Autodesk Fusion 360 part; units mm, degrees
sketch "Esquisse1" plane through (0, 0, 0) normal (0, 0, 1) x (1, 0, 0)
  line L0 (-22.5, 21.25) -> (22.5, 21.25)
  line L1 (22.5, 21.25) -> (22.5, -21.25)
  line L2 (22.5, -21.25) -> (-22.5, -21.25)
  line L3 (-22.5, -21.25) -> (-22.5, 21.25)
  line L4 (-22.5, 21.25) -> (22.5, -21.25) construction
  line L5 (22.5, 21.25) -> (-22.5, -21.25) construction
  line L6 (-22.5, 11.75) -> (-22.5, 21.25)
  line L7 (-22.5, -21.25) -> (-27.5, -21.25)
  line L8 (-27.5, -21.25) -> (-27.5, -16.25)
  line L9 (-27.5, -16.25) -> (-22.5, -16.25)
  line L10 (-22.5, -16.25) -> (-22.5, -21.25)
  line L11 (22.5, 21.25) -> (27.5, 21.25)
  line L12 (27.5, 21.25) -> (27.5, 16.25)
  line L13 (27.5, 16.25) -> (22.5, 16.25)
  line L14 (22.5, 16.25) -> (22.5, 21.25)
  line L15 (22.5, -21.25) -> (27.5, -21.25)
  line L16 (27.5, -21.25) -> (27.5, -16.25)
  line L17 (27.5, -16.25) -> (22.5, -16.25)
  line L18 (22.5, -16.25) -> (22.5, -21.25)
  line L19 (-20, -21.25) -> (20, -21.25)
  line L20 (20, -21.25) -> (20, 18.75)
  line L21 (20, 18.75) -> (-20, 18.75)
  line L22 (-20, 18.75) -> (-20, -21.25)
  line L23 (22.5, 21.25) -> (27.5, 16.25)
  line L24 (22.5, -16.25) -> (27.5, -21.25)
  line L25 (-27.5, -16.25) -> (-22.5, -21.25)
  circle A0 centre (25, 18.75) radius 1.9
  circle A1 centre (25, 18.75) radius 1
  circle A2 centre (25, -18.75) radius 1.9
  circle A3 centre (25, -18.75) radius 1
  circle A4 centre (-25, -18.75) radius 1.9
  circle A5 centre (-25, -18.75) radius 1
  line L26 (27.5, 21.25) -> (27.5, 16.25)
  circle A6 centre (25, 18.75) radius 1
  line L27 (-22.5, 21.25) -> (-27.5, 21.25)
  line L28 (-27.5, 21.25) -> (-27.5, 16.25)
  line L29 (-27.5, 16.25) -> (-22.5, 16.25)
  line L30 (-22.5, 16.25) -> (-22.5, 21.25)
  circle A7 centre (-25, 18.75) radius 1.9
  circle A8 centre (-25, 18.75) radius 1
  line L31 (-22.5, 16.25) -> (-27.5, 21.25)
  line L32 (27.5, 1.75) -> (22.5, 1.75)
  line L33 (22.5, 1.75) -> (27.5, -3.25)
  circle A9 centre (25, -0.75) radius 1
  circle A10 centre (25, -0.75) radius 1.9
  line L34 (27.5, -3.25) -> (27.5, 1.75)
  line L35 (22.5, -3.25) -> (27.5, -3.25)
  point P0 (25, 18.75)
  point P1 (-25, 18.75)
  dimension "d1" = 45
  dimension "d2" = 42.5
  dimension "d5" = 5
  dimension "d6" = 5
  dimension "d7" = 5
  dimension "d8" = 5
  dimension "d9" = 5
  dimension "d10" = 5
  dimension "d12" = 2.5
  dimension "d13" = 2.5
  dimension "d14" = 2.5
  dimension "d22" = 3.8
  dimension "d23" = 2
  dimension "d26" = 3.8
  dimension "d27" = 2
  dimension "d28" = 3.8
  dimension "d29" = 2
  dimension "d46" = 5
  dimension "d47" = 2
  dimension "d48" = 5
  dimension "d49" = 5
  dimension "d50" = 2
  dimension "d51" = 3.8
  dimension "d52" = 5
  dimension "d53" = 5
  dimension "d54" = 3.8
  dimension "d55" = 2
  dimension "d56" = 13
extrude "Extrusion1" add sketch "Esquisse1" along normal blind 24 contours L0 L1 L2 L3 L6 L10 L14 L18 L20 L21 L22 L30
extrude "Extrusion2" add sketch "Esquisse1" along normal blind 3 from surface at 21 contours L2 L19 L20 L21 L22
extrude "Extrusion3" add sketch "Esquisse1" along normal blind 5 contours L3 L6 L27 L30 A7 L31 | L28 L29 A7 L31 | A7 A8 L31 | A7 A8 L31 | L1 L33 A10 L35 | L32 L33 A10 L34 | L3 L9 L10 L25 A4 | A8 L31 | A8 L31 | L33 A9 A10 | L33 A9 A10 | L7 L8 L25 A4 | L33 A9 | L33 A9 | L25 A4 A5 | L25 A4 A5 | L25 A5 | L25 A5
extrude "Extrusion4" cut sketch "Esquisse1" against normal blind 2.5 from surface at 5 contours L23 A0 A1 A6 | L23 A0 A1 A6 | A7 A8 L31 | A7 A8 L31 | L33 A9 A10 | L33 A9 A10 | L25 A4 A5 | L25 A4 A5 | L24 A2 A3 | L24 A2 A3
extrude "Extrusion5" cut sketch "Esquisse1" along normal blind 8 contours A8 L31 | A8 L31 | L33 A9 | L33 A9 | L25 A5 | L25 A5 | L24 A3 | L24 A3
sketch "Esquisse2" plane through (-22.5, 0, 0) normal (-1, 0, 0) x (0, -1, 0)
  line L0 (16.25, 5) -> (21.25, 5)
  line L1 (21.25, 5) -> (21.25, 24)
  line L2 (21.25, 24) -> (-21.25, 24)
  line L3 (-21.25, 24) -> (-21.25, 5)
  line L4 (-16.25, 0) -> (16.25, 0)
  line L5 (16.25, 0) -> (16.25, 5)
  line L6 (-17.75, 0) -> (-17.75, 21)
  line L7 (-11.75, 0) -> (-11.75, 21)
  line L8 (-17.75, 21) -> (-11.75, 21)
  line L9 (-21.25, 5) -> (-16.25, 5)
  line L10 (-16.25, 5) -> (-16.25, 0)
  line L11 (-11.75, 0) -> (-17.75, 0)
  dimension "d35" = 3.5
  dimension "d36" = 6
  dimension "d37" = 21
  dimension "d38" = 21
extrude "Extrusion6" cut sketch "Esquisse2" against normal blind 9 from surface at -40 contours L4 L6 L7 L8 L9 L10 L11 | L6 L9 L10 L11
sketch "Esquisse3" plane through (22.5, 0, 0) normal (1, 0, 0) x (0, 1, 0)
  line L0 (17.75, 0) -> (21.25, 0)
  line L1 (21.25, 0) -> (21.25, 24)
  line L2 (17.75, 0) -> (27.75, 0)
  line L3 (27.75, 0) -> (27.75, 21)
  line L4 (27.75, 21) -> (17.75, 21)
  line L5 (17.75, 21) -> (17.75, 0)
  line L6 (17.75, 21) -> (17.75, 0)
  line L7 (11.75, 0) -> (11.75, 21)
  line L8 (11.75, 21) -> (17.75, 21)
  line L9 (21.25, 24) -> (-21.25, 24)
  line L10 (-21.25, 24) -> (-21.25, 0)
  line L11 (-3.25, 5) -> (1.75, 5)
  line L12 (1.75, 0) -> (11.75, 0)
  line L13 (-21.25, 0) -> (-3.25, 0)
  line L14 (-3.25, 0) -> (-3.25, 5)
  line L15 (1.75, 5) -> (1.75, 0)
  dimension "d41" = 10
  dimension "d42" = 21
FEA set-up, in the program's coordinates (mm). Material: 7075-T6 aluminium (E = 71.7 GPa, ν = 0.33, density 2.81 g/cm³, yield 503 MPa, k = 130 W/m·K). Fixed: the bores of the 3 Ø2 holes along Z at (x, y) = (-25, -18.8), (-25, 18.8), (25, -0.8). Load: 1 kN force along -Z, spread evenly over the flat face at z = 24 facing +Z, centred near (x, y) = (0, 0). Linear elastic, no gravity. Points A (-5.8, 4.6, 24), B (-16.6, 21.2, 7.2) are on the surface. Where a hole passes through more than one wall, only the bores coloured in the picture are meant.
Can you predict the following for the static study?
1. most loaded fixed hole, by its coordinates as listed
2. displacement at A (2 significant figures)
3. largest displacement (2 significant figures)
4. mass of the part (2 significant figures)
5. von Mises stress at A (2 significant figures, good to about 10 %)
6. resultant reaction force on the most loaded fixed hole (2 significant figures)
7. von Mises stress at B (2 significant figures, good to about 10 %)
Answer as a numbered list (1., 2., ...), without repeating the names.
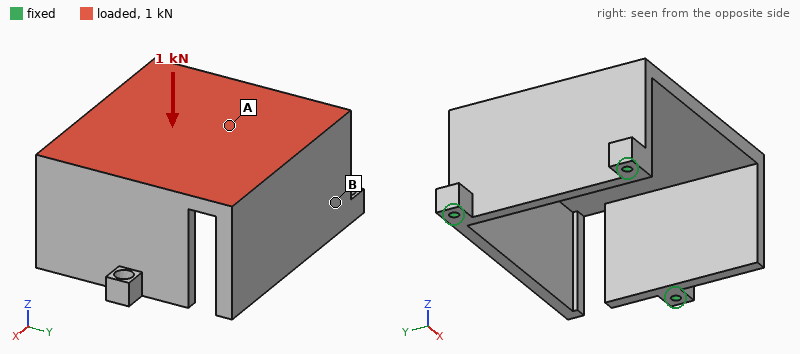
1. (25, -0.8)
2. 37 µm
3. 68 µm
4. 34 g
5. 21 MPa
6. 510 N
7. 7.3 MPa
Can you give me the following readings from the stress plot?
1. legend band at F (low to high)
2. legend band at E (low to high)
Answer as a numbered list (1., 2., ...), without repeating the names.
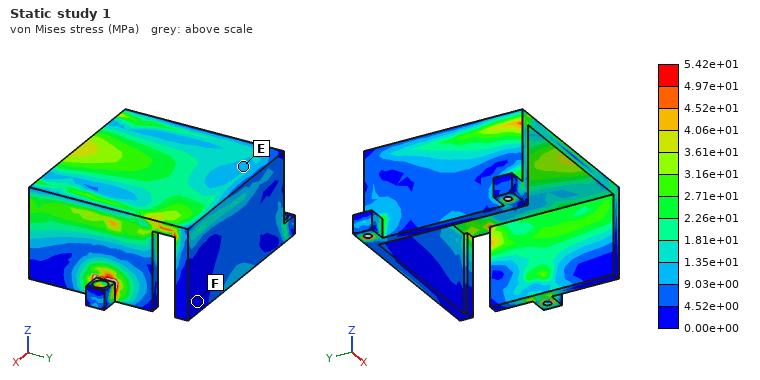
1. 0.00e+00 to 4.52e+00 MPa
2. 9.03e+00 to 1.35e+01 MPa
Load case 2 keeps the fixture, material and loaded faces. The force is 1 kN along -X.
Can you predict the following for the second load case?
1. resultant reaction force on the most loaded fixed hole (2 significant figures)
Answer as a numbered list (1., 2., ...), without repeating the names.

1. 520 N
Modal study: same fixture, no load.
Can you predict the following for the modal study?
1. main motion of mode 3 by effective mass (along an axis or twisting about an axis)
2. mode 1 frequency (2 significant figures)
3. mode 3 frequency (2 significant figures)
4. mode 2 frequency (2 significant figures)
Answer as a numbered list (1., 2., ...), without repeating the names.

1. along Z
2. 2200 Hz
3. 5700 Hz
4. 3400 Hz
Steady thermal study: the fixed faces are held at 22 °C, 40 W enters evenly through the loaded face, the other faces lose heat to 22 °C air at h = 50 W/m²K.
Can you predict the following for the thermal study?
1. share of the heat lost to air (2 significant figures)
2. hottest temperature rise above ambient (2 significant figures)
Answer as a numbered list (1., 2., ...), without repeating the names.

1. 33 %
2. 49 K
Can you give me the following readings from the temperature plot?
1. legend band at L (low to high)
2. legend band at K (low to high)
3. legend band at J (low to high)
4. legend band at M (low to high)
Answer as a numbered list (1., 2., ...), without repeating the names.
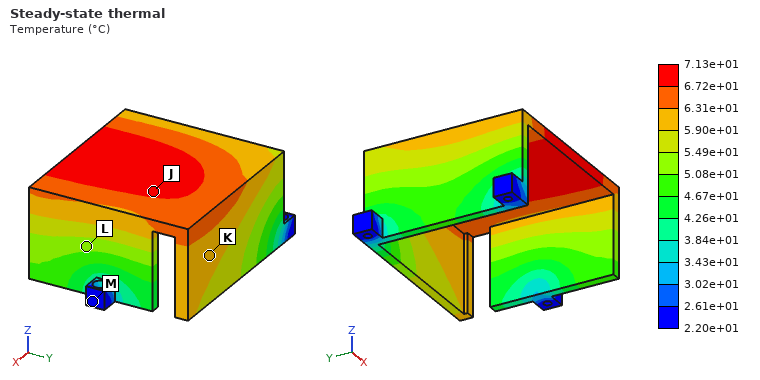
1. 5.08e+01 to 5.49e+01 °C
2. 5.90e+01 to 6.31e+01 °C
3. 6.72e+01 to 7.13e+01 °C
4. 2.20e+01 to 2.61e+01 °C
